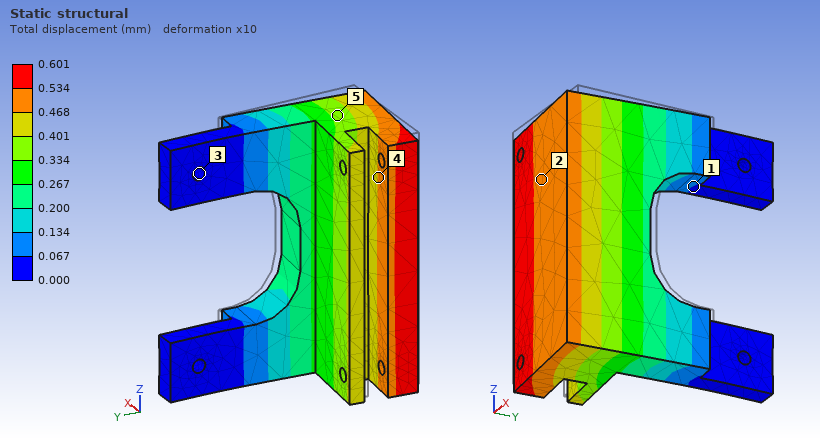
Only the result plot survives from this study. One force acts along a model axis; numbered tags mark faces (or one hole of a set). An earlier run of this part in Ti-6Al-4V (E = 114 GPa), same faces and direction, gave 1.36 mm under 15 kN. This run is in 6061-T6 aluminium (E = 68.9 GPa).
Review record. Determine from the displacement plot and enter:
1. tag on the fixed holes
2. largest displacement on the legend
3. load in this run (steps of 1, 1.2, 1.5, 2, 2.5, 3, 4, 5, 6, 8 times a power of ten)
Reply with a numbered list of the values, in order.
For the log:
1. 3
2. 0.601 mm
3. 4 kN
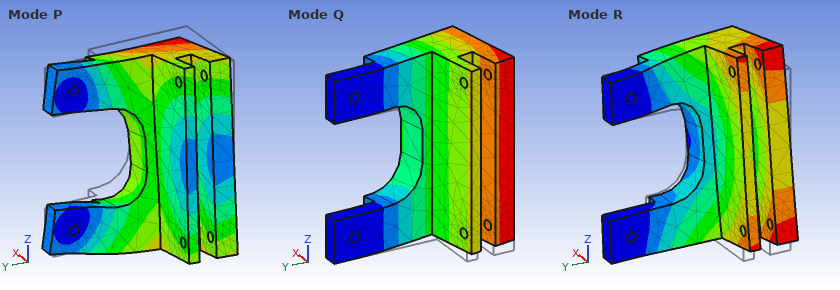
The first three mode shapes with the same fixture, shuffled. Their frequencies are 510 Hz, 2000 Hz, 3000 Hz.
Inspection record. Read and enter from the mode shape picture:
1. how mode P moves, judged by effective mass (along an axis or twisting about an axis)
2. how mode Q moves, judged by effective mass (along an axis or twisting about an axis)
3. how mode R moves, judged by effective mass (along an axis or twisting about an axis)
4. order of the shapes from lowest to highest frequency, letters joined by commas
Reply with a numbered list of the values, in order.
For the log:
1. along Z
2. along X
3. along Z
4. Q, R, P
